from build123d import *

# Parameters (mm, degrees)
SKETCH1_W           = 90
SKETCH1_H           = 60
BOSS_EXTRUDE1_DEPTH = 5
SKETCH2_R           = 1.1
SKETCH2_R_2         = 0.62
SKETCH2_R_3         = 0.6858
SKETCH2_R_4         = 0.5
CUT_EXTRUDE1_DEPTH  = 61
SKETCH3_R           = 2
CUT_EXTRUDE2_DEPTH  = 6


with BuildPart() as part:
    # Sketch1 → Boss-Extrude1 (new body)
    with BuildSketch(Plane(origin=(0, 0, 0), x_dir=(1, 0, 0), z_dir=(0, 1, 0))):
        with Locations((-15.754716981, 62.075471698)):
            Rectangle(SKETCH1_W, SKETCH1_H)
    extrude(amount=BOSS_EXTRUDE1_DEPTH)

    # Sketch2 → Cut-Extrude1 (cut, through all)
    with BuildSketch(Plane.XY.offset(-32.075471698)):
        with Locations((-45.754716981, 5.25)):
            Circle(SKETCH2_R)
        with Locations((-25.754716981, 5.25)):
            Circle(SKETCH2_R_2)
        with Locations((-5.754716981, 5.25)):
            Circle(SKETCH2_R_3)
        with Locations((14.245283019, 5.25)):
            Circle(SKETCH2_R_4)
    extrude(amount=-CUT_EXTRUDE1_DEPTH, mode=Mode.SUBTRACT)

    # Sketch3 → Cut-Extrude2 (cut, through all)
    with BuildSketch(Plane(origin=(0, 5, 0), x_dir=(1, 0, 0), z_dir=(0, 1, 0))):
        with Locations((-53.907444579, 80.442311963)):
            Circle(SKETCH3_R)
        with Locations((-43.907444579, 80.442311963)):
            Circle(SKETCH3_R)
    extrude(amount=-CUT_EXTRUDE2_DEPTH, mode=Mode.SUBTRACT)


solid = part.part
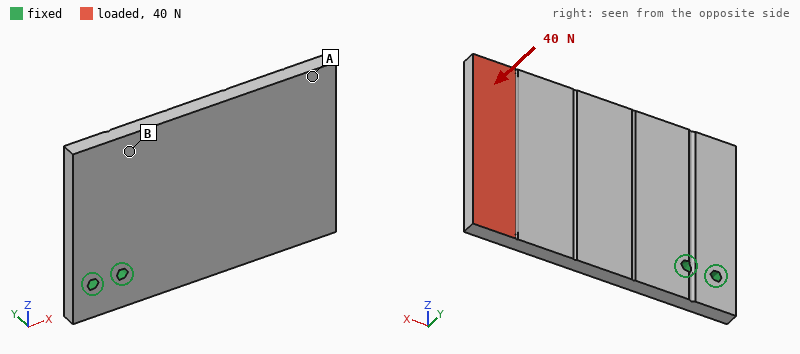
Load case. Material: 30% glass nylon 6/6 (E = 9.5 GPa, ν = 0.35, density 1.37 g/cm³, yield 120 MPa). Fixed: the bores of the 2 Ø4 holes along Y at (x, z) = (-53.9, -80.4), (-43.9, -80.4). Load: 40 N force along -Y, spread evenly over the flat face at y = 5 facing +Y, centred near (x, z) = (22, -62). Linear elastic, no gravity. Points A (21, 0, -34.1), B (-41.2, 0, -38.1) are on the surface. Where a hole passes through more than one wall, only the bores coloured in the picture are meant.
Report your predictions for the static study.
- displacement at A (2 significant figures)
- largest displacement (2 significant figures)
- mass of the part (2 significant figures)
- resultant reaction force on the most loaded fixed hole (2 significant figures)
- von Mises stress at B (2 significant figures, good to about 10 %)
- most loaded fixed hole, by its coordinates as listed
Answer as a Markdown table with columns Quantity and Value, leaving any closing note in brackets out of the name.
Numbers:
| Quantity | Value |
|---|---|
| displacement at A | 1.1 mm |
| largest displacement | 1.2 mm |
| mass of the part | 37 g |
| resultant reaction force on the most loaded fixed hole | 150 N |
| von Mises stress at B | 4.5 MPa |
| most loaded fixed hole, by its coordinates as listed | (-43.9, -80.4) |
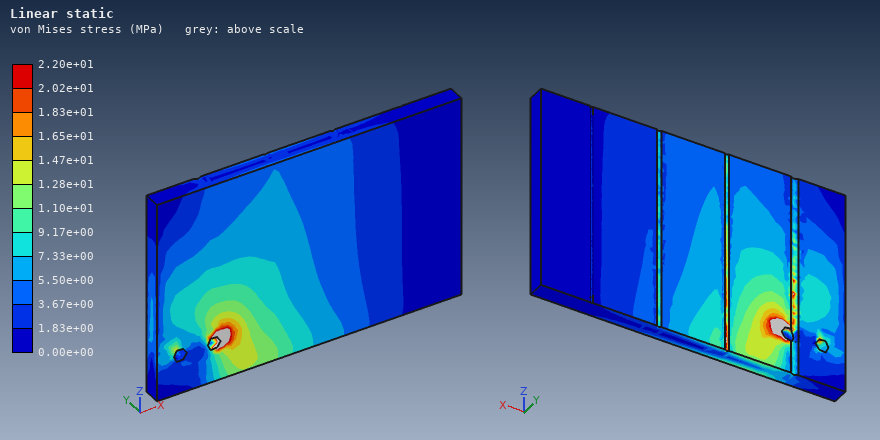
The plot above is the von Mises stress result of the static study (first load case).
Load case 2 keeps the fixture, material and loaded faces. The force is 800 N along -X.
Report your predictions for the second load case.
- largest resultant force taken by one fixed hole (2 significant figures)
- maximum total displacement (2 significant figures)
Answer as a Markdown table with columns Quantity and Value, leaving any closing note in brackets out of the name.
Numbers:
| Quantity | Value |
|---|---|
| largest resultant force taken by one fixed hole | 1.2 kN |
| maximum total displacement | 1.2 mm |
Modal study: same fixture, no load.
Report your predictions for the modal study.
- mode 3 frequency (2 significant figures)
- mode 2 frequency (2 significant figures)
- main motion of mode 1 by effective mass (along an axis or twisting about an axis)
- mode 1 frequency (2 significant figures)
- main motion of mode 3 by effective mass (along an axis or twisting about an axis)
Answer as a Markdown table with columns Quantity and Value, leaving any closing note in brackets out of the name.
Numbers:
| Quantity | Value |
|---|---|
| mode 3 frequency | 1100 Hz |
| mode 2 frequency | 650 Hz |
| main motion of mode 1 by effective mass | along Y |
| mode 1 frequency | 310 Hz |
| main motion of mode 3 by effective mass | along Z |
